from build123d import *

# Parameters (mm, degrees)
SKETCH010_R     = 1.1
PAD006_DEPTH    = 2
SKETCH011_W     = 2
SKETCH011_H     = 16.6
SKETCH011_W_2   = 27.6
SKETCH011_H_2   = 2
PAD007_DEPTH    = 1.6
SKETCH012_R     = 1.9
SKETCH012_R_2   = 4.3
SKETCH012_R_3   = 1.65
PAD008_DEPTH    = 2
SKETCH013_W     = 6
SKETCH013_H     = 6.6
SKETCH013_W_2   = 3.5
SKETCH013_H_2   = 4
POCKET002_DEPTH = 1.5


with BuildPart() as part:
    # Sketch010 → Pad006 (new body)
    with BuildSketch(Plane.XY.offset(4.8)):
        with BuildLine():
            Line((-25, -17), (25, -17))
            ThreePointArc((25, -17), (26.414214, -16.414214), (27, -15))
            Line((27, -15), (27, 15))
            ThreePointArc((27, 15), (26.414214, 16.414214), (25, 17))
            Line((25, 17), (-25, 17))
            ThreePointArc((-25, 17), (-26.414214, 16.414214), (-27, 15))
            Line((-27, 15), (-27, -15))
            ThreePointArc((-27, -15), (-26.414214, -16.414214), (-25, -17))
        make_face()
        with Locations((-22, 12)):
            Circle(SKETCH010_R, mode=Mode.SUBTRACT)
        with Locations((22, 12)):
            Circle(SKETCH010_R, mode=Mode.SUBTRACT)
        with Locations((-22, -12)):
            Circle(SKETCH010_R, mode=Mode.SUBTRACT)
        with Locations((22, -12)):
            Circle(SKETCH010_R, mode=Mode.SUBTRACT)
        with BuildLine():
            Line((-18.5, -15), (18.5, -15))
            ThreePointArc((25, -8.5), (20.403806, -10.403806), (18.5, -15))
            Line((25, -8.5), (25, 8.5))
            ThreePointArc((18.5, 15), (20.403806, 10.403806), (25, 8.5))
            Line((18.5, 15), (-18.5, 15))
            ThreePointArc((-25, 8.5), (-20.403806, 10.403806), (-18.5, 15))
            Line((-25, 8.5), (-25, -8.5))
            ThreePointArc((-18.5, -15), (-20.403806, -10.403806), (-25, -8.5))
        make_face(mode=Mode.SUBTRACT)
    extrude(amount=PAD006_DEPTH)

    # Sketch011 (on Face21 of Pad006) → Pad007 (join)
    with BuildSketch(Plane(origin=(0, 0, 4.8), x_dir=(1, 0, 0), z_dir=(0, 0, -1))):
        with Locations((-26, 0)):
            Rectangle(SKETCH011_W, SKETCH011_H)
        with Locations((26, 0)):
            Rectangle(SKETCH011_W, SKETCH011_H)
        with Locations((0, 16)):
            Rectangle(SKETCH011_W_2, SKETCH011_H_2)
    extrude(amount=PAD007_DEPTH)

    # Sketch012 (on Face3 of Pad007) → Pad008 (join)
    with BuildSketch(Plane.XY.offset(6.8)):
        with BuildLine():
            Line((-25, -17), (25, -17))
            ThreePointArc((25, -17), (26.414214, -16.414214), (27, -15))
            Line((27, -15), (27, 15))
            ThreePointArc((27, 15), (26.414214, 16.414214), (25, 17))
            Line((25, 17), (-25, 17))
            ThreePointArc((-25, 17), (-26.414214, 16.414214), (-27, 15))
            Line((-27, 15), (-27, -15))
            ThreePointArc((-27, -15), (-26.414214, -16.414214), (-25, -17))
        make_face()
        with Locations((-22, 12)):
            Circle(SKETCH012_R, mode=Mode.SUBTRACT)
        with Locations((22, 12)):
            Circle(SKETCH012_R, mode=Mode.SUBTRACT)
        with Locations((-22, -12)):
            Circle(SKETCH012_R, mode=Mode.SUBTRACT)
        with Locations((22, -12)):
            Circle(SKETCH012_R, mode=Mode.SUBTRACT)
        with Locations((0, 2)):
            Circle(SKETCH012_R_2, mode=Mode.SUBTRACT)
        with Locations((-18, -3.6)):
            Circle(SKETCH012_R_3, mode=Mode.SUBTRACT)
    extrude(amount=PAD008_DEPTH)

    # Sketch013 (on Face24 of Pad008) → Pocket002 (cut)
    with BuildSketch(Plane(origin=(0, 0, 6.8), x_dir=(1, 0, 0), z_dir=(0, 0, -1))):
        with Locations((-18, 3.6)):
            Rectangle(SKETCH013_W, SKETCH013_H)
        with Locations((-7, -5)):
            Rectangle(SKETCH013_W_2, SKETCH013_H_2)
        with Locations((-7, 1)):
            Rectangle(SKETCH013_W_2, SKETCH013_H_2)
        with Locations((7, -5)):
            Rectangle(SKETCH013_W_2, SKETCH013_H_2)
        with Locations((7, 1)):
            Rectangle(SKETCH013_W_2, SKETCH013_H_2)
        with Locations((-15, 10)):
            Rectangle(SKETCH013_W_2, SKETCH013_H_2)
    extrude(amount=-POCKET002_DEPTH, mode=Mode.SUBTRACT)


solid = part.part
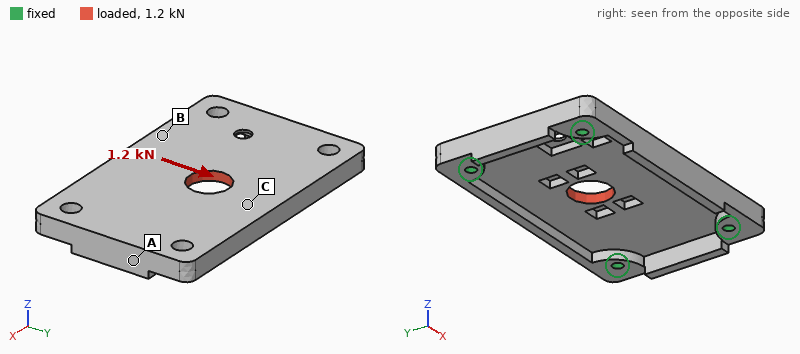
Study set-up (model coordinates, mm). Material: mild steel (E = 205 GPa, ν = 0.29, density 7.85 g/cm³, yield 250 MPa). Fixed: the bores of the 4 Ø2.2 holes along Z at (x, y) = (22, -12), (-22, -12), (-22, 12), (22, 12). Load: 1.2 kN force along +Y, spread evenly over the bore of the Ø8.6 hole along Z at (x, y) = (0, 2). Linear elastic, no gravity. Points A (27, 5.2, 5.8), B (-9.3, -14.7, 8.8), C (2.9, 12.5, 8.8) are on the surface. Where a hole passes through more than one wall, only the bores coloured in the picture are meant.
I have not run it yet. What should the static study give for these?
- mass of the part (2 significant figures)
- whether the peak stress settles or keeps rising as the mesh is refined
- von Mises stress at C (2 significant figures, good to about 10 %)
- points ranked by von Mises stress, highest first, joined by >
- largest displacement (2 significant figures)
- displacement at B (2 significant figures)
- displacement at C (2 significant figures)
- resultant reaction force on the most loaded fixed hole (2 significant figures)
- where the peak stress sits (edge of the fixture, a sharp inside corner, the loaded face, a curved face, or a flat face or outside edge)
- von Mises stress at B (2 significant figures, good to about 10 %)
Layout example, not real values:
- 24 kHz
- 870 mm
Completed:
- 34 g
- keeps rising
- 24 MPa
- C > B > A
- 6.4 µm
- 4.0 µm
- 5.7 µm
- 360 N
- edge of the fixture
- 13 MPa
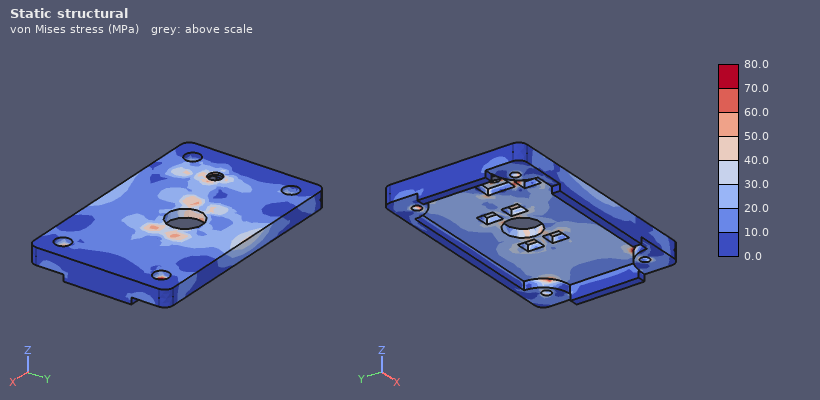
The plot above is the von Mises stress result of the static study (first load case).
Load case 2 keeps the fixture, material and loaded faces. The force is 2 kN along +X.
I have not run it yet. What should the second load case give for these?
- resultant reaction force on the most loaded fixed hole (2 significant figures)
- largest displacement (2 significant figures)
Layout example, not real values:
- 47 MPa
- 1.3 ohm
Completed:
- 560 N
- 5.9 µm
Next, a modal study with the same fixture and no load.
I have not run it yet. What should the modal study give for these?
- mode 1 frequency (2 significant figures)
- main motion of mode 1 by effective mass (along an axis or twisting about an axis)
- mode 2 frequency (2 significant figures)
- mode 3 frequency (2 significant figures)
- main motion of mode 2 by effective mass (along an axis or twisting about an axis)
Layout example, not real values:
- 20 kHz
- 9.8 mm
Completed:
- 6400 Hz
- along Z
- 9000 Hz
- 12 kHz
- twisting about X
